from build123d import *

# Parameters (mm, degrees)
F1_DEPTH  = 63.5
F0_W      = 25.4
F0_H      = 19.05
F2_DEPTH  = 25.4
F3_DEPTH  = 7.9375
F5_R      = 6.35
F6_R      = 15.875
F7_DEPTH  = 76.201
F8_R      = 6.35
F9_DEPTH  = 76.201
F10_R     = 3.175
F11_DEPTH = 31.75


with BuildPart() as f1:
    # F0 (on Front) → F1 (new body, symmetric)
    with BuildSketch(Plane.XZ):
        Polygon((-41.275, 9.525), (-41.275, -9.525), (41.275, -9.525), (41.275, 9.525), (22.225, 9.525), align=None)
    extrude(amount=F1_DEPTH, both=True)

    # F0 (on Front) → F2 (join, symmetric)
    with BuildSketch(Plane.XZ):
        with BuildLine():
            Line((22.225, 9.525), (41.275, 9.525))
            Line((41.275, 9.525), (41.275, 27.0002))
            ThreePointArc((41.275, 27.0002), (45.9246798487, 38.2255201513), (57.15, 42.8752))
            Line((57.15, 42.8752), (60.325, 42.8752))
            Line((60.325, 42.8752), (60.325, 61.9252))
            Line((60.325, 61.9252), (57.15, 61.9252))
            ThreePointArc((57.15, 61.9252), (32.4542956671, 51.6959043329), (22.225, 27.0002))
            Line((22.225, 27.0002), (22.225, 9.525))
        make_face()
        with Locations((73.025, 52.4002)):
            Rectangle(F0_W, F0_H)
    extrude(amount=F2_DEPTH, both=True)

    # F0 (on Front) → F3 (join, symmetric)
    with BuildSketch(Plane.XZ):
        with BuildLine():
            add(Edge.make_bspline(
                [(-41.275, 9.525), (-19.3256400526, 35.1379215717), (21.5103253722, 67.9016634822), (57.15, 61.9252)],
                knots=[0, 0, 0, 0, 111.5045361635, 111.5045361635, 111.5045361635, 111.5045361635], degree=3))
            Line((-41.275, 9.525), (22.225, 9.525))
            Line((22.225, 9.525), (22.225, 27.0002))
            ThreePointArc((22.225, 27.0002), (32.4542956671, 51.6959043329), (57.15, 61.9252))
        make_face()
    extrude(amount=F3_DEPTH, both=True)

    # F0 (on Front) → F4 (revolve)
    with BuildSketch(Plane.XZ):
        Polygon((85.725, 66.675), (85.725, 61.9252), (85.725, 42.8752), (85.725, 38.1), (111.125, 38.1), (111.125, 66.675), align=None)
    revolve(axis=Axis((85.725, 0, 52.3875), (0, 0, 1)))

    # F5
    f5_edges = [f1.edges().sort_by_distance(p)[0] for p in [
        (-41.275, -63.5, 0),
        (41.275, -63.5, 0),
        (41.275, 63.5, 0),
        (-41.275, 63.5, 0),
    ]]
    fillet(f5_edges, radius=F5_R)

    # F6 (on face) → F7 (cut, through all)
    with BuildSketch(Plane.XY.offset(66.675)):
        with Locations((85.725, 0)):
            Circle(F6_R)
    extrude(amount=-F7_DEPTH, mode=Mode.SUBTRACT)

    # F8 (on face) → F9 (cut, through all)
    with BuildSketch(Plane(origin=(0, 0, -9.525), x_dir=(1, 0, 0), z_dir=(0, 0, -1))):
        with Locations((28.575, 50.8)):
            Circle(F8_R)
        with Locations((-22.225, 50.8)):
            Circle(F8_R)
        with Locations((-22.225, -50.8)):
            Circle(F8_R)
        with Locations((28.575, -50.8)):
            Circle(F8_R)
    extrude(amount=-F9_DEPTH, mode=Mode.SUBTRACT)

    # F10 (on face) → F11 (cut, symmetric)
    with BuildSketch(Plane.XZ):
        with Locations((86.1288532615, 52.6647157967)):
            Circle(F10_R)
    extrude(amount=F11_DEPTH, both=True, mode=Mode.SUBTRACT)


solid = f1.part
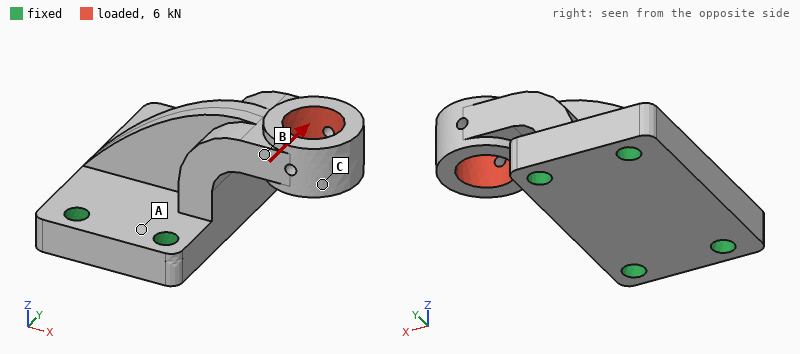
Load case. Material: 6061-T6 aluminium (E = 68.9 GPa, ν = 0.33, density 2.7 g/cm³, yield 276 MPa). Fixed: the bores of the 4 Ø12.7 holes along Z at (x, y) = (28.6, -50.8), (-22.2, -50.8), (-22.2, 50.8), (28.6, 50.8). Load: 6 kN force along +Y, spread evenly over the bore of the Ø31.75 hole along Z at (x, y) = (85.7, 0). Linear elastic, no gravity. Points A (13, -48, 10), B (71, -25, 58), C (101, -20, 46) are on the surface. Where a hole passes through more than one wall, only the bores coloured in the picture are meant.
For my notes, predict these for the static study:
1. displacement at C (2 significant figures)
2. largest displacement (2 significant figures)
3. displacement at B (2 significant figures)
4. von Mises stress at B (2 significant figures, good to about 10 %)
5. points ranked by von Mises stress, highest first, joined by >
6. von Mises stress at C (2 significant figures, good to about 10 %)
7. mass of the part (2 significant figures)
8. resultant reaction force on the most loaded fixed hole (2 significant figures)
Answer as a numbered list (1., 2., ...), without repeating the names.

1. 0.32 mm
2. 0.35 mm
3. 0.20 mm
4. 29 MPa
5. B > C > A
6. 18 MPa
7. 860 g
8. 5.2 kN
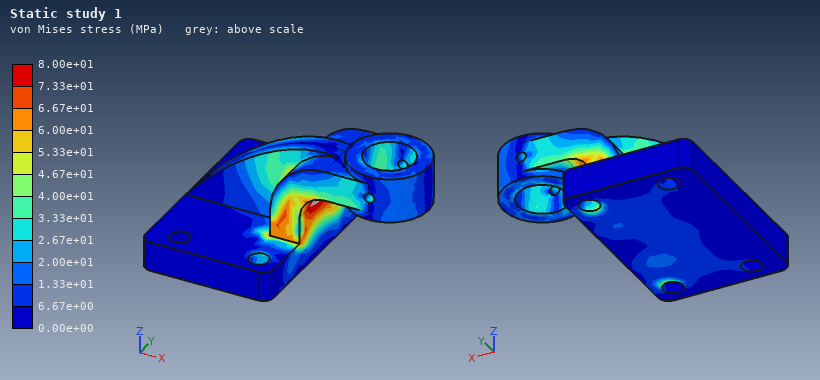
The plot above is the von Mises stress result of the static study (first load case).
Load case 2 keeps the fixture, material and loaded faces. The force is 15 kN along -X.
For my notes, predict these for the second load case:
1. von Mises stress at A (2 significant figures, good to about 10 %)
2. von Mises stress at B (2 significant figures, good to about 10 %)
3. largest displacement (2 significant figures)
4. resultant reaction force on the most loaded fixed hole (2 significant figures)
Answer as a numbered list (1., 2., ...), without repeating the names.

1. 20 MPa
2. 22 MPa
3. 0.35 mm
4. 8.6 kN
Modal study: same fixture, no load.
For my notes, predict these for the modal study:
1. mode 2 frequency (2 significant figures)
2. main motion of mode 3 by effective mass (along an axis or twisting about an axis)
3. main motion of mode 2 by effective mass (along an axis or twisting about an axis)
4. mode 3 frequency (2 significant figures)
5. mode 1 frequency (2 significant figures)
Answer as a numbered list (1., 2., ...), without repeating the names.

1. 2200 Hz
2. along X
3. along Y
4. 4400 Hz
5. 2000 Hz
